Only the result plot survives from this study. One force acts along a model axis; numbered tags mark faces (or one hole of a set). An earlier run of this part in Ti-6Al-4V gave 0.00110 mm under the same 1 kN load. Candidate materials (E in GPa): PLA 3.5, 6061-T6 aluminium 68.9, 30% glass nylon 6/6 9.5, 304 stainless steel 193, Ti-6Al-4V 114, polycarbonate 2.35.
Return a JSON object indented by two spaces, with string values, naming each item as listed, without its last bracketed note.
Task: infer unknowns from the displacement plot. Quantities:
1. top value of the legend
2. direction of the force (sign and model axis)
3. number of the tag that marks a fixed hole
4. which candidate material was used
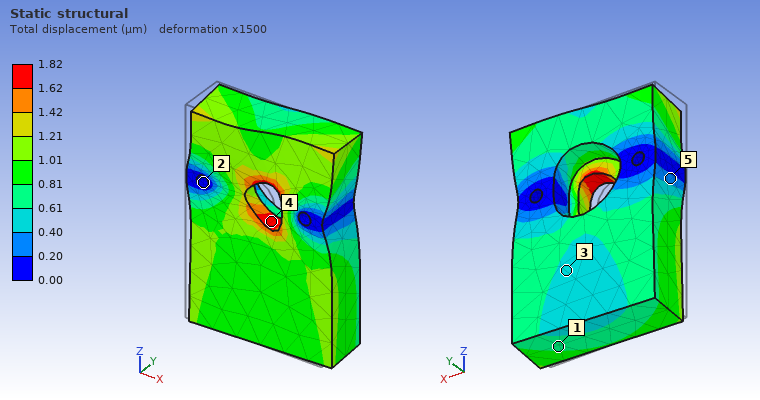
{
  "top value of the legend": "1.82 µm",
  "direction of the force": "+X",
  "number of the tag that marks a fixed hole": "2",
  "which candidate material was used": "6061-T6 aluminium"
}
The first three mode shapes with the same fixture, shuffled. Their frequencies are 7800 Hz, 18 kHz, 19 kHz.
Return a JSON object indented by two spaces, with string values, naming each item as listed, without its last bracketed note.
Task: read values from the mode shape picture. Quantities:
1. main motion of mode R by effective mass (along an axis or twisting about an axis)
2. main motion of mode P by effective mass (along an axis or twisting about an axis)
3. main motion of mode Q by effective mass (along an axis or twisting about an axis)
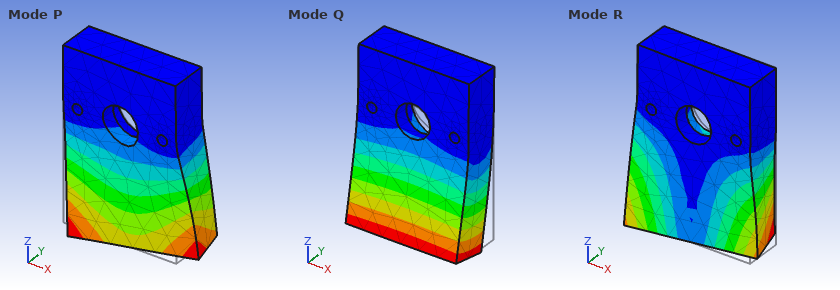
{
  "main motion of mode R by effective mass": "along X",
  "main motion of mode P by effective mass": "along X",
  "main motion of mode Q by effective mass": "along Y"
}
